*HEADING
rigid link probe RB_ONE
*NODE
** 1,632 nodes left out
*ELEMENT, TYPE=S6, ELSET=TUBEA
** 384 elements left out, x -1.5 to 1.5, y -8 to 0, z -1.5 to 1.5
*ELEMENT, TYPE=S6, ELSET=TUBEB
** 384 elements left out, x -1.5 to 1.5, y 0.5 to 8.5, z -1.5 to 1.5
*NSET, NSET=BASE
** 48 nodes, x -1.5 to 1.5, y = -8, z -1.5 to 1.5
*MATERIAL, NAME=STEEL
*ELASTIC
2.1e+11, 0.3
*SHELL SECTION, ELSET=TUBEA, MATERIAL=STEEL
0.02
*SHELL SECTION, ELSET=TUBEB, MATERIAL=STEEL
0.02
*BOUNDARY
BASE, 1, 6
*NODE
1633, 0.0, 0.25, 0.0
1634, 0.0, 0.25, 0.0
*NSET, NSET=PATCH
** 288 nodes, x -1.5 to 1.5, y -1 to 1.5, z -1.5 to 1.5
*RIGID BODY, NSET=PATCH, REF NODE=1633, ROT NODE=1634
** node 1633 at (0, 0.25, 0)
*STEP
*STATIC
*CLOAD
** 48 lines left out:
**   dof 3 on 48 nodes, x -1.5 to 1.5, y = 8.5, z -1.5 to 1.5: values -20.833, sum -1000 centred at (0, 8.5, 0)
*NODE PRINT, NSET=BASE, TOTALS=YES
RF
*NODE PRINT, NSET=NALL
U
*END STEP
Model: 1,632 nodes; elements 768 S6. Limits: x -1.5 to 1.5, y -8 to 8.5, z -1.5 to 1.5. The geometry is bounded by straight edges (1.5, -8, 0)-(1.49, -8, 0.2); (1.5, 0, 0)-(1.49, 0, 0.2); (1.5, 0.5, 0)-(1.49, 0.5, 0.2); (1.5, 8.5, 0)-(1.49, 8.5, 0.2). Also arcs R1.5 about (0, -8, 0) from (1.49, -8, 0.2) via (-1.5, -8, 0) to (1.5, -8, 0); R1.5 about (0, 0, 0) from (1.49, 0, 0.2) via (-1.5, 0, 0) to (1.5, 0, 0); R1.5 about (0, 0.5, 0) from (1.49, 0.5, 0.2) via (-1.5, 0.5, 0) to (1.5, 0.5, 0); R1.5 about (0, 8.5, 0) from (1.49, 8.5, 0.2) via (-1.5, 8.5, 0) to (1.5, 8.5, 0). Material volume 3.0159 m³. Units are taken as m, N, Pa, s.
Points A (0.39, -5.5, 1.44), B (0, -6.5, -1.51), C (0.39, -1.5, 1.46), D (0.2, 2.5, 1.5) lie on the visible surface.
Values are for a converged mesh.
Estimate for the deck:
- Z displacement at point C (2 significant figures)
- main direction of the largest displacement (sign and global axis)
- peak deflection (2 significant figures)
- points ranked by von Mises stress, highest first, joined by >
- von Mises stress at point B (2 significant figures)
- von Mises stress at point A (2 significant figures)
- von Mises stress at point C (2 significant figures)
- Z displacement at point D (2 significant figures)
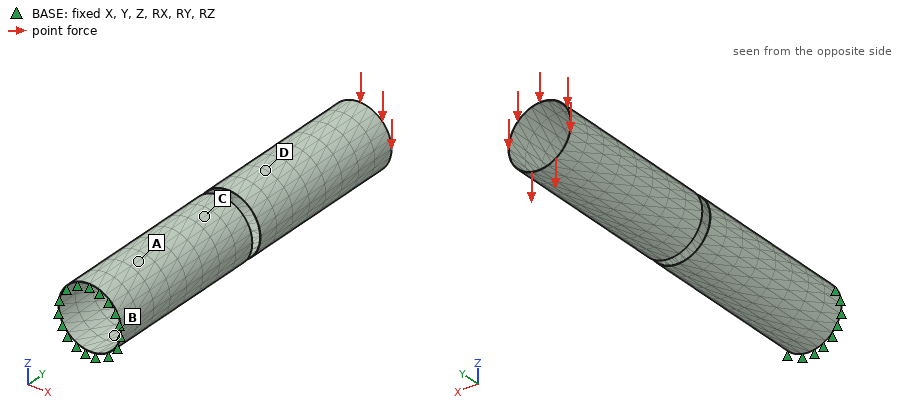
-7.7e-06 m
-Z
3.2e-05 m
B > A > C > D
1.1e+05 Pa
95000 Pa
68000 Pa
-1.6e-05 m
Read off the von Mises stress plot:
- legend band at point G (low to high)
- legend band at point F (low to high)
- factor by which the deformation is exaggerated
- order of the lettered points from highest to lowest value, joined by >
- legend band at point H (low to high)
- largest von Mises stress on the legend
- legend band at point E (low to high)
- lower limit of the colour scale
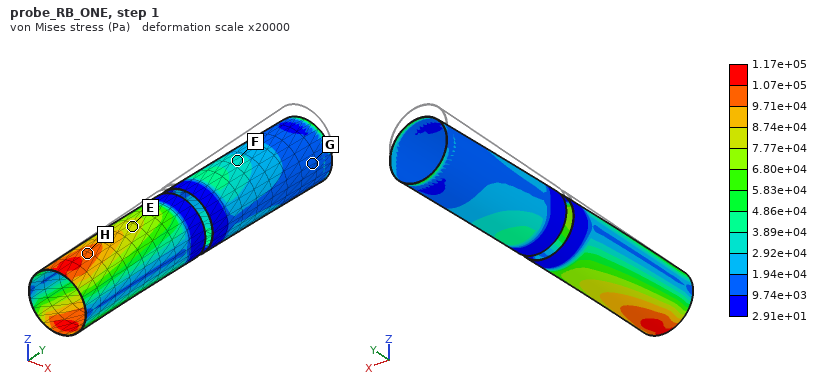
9.74e+03 to 1.94e+04 Pa
2.92e+04 to 3.89e+04 Pa
20000
H > E > F > G
9.71e+04 to 1.07e+05 Pa
1.17e+05 Pa
7.77e+04 to 8.74e+04 Pa
2.91e+01 Pa
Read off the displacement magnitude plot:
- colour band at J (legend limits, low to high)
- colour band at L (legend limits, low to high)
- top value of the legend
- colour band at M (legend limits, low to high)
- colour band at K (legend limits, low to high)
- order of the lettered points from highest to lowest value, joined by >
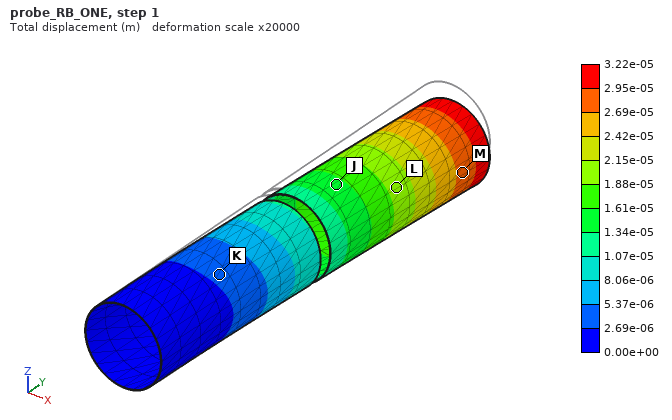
1.34e-05 to 1.61e-05 m
1.88e-05 to 2.15e-05 m
3.22e-05 m
2.69e-05 to 2.95e-05 m
2.69e-06 to 5.37e-06 m
M > L > J > K
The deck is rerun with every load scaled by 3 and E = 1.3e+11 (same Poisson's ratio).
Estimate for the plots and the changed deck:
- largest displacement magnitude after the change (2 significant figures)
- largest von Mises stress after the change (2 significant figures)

1.6e-04 m
3.5e+05 Pa
